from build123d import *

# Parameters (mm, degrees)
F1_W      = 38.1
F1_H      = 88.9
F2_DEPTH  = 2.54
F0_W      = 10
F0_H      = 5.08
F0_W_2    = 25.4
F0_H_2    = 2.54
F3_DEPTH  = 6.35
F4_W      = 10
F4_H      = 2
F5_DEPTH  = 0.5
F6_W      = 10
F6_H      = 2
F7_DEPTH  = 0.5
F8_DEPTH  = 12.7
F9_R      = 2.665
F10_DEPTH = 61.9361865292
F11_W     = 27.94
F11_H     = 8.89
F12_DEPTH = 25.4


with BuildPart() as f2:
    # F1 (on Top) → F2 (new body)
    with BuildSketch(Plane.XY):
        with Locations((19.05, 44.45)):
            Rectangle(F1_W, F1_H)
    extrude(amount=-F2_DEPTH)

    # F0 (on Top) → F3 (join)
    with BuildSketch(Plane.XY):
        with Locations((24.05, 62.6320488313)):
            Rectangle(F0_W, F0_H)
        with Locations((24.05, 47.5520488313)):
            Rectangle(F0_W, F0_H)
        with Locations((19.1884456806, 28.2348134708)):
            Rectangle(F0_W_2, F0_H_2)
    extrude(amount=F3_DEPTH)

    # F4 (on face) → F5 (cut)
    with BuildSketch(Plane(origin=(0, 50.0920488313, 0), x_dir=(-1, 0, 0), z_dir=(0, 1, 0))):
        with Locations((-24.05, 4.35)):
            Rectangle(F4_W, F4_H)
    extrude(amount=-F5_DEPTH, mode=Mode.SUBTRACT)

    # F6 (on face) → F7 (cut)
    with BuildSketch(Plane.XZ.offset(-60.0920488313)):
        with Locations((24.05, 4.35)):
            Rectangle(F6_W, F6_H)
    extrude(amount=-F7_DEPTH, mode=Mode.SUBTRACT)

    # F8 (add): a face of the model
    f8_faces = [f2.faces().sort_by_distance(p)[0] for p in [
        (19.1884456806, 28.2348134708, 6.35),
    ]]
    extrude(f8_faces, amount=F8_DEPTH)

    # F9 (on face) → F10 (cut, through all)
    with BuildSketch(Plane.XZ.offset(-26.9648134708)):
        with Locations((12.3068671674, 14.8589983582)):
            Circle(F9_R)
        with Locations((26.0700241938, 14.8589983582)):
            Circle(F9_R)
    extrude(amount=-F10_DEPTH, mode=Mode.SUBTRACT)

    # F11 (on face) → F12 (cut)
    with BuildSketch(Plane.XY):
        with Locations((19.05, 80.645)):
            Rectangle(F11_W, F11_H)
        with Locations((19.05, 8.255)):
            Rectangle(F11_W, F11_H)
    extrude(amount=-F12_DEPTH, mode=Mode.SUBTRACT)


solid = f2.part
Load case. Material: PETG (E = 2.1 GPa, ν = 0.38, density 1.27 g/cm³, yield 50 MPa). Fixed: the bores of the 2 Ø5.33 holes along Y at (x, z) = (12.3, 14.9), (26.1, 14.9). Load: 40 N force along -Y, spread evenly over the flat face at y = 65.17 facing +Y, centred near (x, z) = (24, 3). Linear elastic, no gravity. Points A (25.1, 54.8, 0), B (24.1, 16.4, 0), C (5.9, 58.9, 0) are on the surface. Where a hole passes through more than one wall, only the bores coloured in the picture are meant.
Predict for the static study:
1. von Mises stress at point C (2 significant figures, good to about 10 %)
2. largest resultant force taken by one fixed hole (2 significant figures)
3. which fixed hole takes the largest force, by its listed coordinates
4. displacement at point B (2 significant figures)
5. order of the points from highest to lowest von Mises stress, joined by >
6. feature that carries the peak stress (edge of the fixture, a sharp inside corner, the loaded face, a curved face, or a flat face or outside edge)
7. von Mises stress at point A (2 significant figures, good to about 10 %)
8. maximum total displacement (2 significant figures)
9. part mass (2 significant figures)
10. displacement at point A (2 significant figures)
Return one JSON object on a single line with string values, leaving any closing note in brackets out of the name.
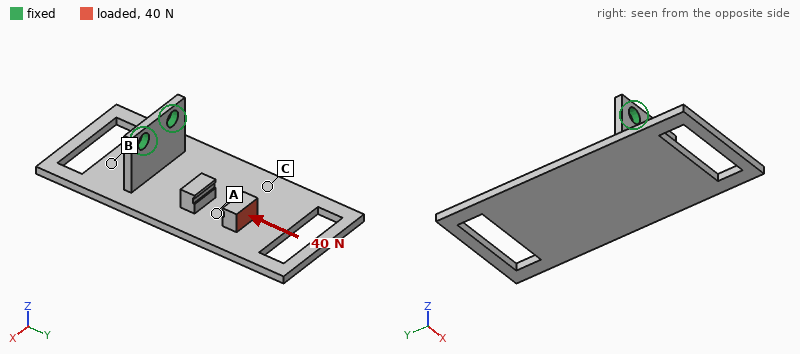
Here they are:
{"von Mises stress at point C": "2.7 MPa", "largest resultant force taken by one fixed hole": "31 N", "which fixed hole takes the largest force, by its listed coordinates": "(26.1, 14.9)", "displacement at point B": "0.41 mm", "order of the points from highest to lowest von Mises stress, joined by >": "A > C > B", "feature that carries the peak stress": "a flat face or outside edge", "von Mises stress at point A": "5.7 MPa", "maximum total displacement": "1.2 mm", "part mass": "12 g", "displacement at point A": "0.45 mm"}
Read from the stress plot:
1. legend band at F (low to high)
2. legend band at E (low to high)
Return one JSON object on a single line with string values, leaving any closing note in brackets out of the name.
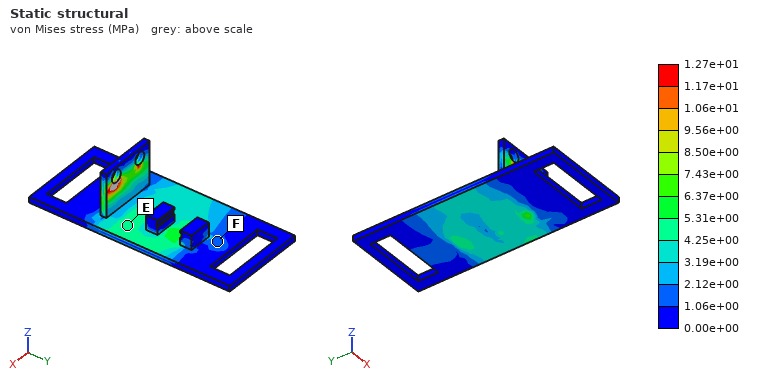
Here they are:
{"legend band at F": "1.06e+00 to 2.12e+00 MPa", "legend band at E": "4.25e+00 to 5.31e+00 MPa"}
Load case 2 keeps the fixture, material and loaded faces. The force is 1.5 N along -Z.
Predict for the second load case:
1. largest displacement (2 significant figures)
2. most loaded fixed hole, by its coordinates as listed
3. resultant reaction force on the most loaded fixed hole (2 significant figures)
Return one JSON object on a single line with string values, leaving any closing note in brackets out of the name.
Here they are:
{"largest displacement": "1.00 mm", "most loaded fixed hole, by its coordinates as listed": "(26.1, 14.9)", "resultant reaction force on the most loaded fixed hole": "1.2 N"}
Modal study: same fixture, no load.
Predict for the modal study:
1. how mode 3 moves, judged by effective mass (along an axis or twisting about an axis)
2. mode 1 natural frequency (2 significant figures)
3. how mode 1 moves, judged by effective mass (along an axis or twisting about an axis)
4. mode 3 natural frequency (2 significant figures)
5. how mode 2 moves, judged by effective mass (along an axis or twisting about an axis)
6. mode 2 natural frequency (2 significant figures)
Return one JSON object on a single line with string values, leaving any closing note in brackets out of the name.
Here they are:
{"how mode 3 moves, judged by effective mass": "along Y", "mode 1 natural frequency": "110 Hz", "how mode 1 moves, judged by effective mass": "along Z", "mode 3 natural frequency": "440 Hz", "how mode 2 moves, judged by effective mass": "along X", "mode 2 natural frequency": "230 Hz"}
